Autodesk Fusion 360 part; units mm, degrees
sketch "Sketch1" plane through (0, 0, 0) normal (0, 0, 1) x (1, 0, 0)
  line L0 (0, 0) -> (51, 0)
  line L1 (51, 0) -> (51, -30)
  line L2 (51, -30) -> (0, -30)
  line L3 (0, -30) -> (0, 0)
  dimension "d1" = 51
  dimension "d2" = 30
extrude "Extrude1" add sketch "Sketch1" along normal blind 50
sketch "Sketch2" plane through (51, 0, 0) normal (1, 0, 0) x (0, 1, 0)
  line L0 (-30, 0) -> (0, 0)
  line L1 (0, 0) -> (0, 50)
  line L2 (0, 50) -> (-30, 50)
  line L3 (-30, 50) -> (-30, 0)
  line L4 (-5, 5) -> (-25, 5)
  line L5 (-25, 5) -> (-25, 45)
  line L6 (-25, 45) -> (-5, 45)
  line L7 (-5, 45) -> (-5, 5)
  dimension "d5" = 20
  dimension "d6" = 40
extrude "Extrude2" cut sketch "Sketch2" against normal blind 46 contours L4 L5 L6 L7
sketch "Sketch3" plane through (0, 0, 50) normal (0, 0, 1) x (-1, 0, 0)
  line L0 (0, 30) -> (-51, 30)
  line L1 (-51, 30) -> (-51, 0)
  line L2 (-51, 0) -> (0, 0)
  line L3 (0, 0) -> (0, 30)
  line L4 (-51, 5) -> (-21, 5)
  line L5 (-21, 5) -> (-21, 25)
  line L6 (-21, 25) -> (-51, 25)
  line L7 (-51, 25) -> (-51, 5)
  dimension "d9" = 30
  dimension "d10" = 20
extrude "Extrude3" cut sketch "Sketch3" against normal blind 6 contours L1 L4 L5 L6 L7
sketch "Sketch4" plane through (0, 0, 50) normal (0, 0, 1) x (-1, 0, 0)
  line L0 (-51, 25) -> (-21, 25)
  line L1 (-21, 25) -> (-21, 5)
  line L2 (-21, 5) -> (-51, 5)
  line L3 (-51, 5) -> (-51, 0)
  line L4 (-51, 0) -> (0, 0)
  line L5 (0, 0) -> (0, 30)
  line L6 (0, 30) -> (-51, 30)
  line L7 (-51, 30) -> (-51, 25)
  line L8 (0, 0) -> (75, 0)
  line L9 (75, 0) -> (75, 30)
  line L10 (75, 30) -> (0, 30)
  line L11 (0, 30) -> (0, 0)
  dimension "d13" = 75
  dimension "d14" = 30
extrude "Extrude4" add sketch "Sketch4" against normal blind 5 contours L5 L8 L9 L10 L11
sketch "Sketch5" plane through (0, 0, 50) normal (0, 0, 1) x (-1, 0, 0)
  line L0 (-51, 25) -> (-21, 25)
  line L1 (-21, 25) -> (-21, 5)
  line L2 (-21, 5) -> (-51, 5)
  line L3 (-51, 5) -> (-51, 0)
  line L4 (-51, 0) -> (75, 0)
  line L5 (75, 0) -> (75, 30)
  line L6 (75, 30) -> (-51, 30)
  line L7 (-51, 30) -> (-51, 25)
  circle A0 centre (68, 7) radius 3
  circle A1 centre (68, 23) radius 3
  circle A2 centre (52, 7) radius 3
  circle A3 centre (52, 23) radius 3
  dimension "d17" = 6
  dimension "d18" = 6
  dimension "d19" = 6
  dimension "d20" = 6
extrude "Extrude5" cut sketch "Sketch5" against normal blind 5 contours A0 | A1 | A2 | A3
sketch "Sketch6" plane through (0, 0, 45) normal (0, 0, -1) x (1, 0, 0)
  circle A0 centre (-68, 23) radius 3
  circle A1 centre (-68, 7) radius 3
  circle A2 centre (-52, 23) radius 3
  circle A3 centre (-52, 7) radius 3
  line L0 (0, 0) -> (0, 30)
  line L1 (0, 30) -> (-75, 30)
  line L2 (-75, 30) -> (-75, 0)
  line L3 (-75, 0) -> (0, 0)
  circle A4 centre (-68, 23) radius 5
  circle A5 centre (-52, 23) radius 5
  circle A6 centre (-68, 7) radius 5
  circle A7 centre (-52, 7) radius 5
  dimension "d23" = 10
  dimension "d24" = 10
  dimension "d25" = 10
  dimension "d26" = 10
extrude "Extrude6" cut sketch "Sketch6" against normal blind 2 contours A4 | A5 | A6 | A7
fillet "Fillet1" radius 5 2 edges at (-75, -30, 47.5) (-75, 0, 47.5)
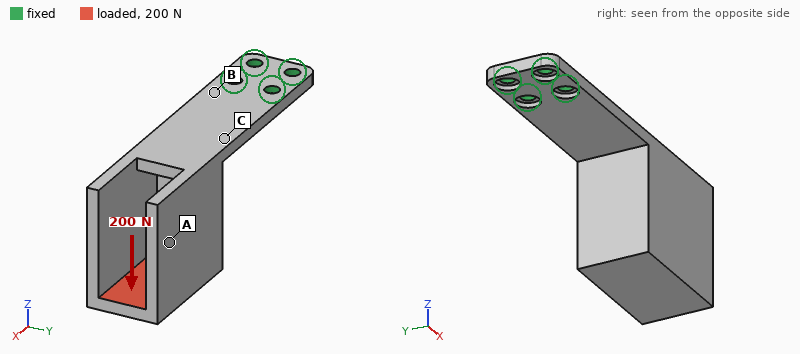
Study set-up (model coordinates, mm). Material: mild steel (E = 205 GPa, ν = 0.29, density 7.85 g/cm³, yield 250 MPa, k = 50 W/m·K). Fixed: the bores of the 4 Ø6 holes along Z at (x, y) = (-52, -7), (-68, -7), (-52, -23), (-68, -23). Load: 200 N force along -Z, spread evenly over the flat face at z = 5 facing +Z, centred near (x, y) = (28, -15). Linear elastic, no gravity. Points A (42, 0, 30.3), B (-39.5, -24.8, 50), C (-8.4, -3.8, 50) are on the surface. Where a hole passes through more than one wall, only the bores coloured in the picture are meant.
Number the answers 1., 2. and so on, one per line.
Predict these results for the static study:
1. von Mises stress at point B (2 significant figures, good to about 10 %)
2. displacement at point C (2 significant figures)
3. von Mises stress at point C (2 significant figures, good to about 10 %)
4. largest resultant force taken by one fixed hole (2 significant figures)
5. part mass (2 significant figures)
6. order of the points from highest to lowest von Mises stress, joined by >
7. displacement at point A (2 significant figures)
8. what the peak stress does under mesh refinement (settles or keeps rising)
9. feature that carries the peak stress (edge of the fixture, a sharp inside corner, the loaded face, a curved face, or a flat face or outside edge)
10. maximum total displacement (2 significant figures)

1. 100 MPa
2. 0.22 mm
3. 59 MPa
4. 410 N
5. 370 g
6. B > C > A
7. 0.72 mm
8. keeps rising
9. edge of the fixture
10. 0.91 mm
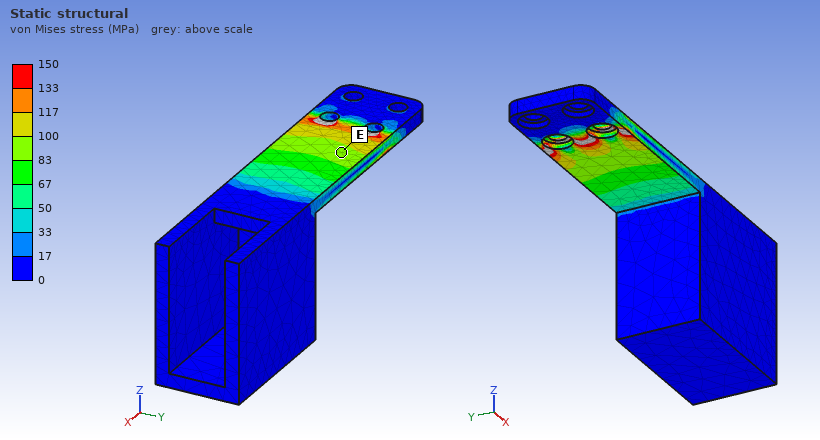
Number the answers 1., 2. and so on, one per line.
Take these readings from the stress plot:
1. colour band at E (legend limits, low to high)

1. 83 to 100 MPa
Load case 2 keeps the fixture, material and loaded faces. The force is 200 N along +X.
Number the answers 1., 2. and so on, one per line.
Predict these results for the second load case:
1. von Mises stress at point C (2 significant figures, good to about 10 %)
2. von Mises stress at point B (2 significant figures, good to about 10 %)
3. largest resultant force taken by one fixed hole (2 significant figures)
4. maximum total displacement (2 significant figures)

1. 67 MPa
2. 65 MPa
3. 210 N
4. 0.69 mm
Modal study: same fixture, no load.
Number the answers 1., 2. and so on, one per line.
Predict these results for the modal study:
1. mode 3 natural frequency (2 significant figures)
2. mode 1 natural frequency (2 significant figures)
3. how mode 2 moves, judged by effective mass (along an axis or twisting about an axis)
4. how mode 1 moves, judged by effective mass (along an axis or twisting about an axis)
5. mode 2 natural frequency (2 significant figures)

1. 1000 Hz
2. 170 Hz
3. along Y
4. along Z
5. 420 Hz
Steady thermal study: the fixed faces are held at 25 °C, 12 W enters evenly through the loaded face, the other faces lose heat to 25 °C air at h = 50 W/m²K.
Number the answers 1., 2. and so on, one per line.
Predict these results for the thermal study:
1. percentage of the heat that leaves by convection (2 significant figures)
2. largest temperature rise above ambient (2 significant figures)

1. 92 %
2. 23 K
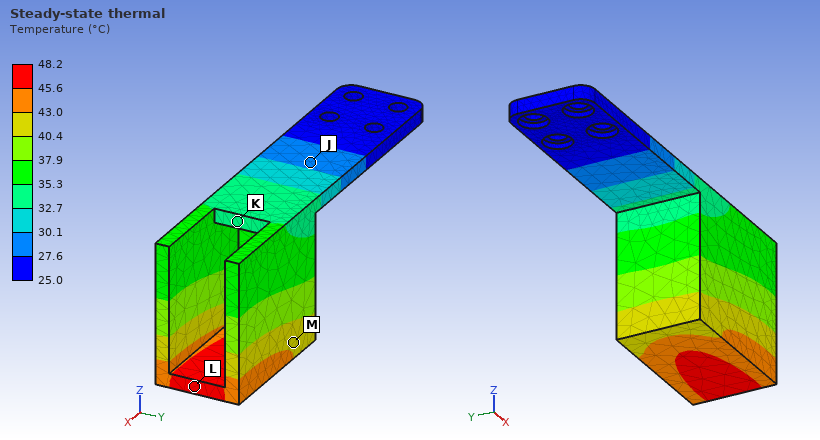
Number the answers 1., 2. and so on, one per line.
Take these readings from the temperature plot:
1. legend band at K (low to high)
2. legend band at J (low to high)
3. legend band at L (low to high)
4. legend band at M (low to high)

1. 32.7 to 35.3 °C
2. 27.6 to 30.1 °C
3. 45.6 to 48.2 °C
4. 40.4 to 43.0 °C
